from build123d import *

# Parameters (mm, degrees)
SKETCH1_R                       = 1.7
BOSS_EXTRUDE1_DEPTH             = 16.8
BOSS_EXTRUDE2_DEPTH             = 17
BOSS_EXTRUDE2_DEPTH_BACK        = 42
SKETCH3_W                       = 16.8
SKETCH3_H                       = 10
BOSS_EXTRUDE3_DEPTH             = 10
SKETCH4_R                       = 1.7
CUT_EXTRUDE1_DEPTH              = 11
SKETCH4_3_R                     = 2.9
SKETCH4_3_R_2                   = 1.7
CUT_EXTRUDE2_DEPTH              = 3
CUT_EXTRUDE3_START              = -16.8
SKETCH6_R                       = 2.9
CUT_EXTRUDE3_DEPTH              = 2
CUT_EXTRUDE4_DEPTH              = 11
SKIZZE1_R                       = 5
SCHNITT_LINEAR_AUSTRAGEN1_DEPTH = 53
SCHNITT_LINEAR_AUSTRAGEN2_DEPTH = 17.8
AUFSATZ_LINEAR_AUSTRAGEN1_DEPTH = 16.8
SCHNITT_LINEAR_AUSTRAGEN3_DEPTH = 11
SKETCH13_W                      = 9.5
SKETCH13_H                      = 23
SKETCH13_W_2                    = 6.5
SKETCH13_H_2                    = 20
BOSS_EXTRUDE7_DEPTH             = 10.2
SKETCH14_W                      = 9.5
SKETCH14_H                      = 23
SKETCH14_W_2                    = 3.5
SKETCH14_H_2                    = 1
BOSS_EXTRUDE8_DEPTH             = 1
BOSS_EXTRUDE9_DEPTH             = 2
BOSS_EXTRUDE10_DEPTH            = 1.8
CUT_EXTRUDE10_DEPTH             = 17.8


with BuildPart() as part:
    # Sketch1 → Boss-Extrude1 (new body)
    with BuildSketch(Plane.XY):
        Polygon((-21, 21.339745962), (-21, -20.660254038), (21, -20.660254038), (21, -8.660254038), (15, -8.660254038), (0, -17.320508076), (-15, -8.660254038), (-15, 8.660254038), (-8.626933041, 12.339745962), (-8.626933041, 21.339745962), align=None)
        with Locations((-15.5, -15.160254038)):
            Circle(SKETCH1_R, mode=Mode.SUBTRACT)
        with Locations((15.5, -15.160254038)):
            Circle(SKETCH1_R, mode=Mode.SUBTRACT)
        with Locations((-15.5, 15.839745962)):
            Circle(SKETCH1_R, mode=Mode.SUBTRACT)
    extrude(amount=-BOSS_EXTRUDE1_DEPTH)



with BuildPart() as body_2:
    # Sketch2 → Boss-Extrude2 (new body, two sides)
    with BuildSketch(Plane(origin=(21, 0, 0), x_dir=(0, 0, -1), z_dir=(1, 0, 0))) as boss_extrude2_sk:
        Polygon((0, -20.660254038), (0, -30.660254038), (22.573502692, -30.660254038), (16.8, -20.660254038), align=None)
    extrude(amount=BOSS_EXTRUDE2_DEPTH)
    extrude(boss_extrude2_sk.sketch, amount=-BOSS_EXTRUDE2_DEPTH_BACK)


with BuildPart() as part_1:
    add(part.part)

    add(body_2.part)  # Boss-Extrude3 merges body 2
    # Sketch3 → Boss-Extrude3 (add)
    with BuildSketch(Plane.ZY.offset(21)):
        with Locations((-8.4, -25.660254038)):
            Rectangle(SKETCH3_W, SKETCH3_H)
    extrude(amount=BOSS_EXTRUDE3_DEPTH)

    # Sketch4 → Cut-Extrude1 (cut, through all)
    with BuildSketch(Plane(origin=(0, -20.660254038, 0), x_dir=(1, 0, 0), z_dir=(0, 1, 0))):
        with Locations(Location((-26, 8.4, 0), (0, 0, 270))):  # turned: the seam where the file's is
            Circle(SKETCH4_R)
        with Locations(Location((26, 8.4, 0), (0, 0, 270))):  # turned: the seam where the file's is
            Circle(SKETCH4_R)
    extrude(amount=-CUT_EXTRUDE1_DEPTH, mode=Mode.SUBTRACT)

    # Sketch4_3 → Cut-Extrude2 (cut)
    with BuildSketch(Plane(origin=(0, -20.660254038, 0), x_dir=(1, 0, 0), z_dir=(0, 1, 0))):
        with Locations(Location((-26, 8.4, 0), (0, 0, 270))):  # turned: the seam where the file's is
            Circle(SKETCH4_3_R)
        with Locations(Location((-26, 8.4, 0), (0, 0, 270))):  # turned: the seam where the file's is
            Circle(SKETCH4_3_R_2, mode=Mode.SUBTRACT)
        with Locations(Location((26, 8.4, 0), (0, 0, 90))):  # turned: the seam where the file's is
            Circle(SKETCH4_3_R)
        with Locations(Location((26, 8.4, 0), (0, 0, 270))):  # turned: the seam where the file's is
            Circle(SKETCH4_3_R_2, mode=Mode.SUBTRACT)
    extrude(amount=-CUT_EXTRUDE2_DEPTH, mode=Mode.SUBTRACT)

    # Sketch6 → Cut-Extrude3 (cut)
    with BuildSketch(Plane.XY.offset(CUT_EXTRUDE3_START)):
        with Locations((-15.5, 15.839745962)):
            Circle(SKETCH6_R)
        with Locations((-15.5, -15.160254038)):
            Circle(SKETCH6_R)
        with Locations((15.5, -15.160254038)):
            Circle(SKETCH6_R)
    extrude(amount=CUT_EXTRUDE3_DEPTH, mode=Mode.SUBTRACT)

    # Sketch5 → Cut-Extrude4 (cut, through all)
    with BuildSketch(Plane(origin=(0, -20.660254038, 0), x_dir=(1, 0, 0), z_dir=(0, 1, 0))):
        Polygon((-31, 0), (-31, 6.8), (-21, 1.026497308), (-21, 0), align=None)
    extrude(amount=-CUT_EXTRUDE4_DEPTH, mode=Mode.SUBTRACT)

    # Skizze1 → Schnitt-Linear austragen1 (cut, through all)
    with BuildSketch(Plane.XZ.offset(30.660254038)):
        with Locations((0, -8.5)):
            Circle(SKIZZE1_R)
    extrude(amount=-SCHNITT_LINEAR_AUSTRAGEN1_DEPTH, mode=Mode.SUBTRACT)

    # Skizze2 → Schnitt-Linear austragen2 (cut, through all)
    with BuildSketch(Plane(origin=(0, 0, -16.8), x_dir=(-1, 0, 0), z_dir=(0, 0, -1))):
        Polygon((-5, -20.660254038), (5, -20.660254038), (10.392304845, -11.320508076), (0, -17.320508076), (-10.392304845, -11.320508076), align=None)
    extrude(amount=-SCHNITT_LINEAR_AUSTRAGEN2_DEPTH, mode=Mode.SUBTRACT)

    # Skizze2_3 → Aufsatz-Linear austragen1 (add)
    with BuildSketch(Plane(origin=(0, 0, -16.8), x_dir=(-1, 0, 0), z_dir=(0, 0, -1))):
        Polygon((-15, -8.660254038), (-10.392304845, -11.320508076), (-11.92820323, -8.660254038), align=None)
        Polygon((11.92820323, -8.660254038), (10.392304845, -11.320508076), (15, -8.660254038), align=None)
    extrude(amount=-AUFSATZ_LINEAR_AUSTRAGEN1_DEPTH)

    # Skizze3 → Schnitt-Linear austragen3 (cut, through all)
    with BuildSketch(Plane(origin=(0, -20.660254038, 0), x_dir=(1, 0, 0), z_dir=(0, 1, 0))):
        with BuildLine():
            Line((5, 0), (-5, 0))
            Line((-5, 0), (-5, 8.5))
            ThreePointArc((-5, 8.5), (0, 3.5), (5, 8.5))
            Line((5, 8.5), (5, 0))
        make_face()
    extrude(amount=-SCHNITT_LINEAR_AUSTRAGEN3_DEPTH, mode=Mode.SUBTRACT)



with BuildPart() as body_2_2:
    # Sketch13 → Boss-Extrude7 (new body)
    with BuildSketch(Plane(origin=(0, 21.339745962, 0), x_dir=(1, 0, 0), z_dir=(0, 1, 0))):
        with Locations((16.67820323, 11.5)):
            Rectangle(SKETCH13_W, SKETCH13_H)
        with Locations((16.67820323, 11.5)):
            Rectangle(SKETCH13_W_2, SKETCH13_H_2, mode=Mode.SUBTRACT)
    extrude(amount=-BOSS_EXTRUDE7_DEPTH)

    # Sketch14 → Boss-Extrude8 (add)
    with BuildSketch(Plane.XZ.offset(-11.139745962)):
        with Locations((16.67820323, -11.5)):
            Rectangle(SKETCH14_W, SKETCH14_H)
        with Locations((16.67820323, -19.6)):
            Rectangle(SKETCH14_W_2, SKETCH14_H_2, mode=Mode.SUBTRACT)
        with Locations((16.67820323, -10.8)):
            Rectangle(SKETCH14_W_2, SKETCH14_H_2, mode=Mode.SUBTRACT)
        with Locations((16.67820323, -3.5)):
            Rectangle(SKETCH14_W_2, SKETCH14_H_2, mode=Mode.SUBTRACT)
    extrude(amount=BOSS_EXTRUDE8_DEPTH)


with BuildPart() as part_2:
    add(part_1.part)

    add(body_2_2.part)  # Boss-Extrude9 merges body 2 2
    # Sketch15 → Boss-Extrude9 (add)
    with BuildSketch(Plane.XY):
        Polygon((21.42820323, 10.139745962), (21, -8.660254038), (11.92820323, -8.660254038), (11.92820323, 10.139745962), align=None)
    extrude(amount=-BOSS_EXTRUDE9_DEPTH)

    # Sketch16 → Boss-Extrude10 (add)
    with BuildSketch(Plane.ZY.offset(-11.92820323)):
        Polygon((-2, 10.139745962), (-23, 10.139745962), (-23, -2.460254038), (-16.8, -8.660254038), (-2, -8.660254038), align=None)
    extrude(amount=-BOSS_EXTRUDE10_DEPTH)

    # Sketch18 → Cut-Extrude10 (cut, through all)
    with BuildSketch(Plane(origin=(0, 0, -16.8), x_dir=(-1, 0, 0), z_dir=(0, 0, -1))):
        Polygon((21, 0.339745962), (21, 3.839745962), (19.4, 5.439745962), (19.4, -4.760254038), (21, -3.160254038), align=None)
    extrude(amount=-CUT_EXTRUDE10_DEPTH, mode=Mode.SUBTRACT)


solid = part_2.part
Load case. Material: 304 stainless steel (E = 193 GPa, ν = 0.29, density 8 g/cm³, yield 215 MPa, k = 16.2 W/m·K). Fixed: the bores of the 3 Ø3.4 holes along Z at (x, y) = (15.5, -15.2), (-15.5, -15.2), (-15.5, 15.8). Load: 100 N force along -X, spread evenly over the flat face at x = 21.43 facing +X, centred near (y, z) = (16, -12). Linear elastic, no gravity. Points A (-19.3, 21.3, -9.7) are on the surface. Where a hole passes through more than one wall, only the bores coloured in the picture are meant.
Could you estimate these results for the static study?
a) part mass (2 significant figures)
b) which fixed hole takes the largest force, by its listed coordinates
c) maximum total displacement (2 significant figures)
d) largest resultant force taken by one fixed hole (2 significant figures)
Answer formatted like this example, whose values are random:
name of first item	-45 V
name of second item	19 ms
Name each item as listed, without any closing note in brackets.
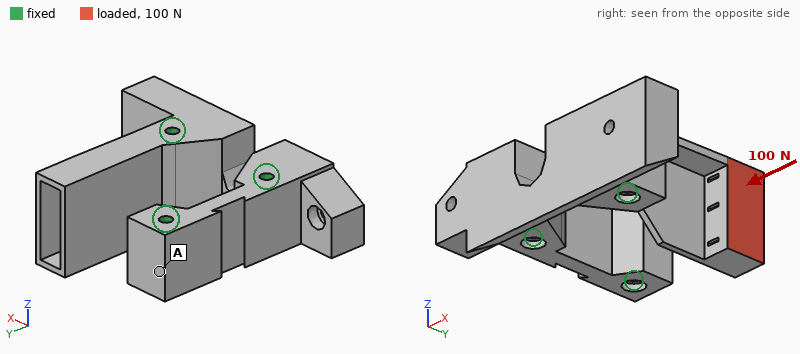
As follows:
part mass	180 g
which fixed hole takes the largest force, by its listed coordinates	(15.5, -15.2)
maximum total displacement	82 µm
largest resultant force taken by one fixed hole	160 N
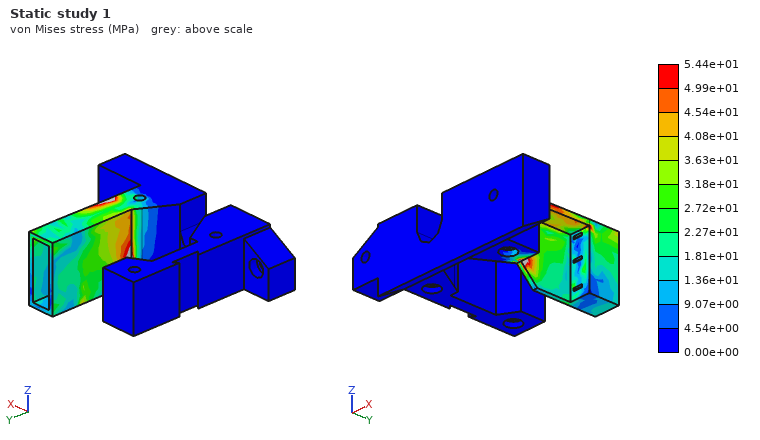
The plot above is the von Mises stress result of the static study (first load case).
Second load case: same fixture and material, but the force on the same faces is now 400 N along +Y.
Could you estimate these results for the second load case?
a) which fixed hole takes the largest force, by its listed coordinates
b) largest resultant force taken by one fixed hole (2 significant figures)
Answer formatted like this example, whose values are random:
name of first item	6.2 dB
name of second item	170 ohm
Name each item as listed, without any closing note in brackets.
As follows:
which fixed hole takes the largest force, by its listed coordinates	(15.5, -15.2)
largest resultant force taken by one fixed hole	420 N
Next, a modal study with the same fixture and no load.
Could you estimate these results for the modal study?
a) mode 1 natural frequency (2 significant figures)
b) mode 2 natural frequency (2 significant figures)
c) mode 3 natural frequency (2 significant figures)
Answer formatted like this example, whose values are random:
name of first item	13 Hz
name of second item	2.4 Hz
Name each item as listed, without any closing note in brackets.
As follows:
mode 1 natural frequency	2200 Hz
mode 2 natural frequency	4500 Hz
mode 3 natural frequency	8400 Hz
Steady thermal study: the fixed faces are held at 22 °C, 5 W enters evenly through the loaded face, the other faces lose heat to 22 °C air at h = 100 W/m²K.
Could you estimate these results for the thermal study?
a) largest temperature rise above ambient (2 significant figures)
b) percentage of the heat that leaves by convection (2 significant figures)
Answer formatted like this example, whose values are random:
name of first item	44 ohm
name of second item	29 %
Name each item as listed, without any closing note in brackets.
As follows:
largest temperature rise above ambient	57 K
percentage of the heat that leaves by convection	93 %
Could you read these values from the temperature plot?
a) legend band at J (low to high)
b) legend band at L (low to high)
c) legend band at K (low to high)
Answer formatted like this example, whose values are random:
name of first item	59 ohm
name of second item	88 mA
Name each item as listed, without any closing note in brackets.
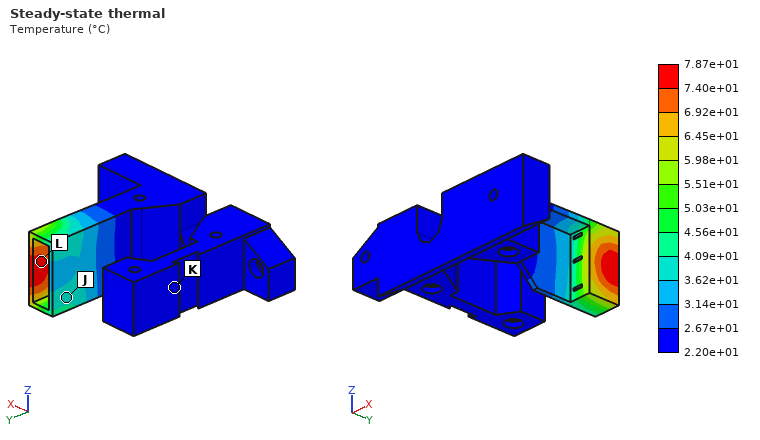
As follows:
legend band at J	3.62e+01 to 4.09e+01 °C
legend band at L	7.40e+01 to 7.87e+01 °C
legend band at K	2.20e+01 to 2.67e+01 °C
